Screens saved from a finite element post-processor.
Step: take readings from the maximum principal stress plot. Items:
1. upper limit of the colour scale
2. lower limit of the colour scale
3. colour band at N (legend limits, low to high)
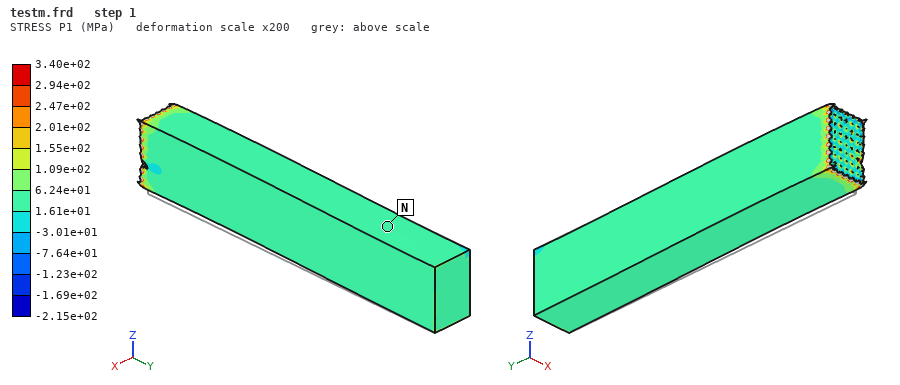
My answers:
3.40e+02 MPa
-2.15e+02 MPa
1.61e+01 to 6.24e+01 MPa
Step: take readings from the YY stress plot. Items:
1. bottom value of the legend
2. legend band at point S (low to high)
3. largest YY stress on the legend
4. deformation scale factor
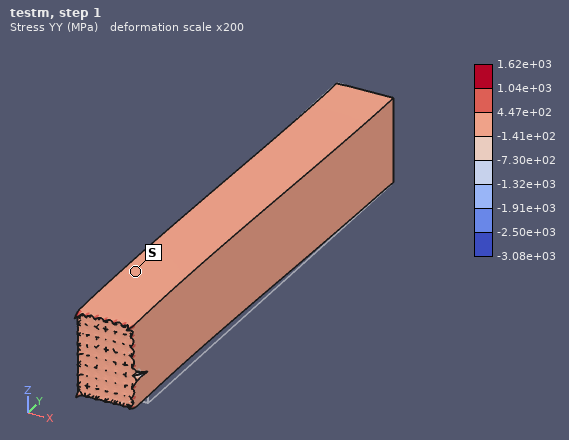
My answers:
-3.08e+03 MPa
-1.41e+02 to 4.47e+02 MPa
1.62e+03 MPa
200
